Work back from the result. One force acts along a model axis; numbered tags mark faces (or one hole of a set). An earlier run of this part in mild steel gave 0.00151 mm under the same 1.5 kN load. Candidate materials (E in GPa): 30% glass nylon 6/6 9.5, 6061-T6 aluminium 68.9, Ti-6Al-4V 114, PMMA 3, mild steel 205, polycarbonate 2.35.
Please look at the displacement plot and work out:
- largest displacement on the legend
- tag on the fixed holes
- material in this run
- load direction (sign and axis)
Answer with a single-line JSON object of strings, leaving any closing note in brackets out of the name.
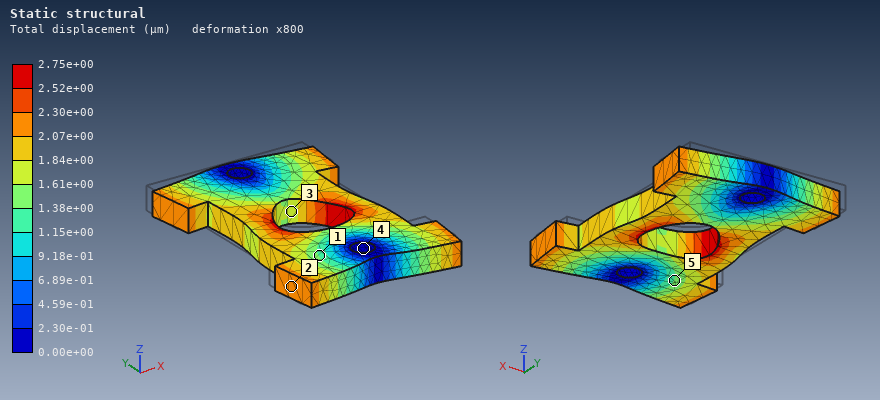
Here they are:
{"largest displacement on the legend": "2.75e+00 µm", "tag on the fixed holes": "4", "material in this run": "Ti-6Al-4V", "load direction": "-Y"}
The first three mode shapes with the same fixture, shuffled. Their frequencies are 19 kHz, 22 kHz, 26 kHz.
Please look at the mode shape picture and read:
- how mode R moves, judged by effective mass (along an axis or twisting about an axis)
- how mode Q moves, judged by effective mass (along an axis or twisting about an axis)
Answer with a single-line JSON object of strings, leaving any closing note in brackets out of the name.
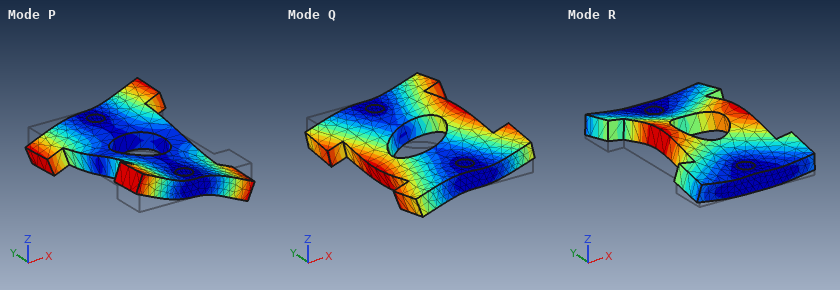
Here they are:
{"how mode R moves, judged by effective mass": "along Z", "how mode Q moves, judged by effective mass": "twisting about Y"}
